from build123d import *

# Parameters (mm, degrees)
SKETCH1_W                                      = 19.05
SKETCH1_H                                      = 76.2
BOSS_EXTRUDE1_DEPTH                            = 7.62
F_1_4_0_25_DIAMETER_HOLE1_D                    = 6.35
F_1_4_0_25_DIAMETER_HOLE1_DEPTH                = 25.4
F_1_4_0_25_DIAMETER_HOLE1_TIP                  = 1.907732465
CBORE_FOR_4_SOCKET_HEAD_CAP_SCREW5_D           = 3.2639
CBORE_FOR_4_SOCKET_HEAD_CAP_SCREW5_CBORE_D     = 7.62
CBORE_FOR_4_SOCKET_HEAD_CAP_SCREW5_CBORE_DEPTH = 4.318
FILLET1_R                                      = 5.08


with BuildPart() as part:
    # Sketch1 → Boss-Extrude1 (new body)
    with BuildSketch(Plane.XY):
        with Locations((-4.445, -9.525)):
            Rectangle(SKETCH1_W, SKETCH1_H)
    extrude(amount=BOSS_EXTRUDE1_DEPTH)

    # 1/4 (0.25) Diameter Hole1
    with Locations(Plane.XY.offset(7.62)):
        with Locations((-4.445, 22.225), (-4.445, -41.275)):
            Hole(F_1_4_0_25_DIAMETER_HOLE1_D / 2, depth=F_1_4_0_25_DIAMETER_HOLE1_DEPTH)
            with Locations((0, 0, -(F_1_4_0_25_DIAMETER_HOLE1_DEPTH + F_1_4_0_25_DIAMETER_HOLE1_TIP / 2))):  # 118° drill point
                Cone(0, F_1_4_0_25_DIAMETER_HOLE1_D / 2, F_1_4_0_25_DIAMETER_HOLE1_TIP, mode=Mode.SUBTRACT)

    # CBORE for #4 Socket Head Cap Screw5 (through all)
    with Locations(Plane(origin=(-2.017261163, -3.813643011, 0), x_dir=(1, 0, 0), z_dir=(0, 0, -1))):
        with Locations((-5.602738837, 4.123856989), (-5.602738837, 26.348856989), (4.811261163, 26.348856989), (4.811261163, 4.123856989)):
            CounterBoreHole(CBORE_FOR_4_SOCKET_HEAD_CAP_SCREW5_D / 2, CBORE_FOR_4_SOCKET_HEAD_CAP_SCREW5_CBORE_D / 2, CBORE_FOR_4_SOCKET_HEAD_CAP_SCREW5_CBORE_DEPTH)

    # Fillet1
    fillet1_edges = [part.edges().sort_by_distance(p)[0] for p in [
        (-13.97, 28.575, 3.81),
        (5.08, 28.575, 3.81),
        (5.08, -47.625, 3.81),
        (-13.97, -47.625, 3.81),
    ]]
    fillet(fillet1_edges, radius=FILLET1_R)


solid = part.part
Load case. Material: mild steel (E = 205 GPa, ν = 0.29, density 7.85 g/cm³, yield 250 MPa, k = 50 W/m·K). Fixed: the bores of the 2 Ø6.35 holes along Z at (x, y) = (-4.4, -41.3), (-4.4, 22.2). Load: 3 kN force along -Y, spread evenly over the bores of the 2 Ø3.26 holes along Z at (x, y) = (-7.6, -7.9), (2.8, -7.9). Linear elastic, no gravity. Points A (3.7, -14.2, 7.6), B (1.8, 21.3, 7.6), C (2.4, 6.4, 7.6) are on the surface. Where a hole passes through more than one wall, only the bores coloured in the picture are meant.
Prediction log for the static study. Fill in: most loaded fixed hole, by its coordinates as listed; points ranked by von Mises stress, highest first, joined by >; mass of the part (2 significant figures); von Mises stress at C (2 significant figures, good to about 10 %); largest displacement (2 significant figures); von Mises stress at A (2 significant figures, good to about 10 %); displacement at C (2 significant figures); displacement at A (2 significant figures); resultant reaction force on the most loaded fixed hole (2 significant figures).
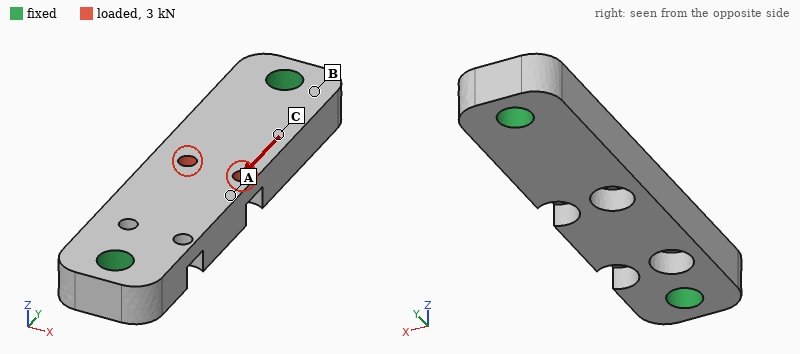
(-4.4, 22.2)
A > C > B
75 g
22 MPa
3.9 µm
35 MPa
1.2 µm
2.9 µm
1.7 kN
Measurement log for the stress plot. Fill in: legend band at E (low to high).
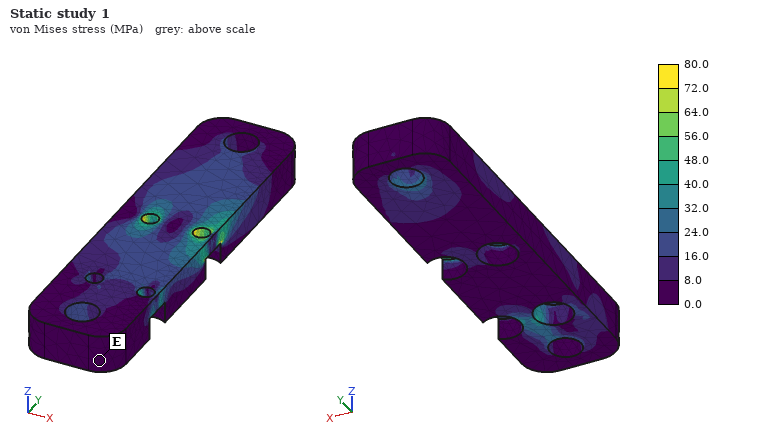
0.0 to 8.0 MPa
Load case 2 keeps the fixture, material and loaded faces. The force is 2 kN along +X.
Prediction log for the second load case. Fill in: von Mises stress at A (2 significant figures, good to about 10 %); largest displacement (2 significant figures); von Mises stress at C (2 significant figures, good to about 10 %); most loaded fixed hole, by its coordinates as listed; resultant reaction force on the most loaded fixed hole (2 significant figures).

28 MPa
14 µm
19 MPa
(-4.4, 22.2)
1.1 kN
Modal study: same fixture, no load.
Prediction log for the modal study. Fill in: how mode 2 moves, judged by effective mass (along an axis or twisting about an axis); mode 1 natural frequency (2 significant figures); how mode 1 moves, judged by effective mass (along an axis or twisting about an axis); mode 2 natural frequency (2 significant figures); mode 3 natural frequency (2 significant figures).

along X
9200 Hz
along Z
14 kHz
16 kHz
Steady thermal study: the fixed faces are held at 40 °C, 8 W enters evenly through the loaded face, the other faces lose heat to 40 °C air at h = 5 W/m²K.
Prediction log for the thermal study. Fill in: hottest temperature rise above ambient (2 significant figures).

28 K
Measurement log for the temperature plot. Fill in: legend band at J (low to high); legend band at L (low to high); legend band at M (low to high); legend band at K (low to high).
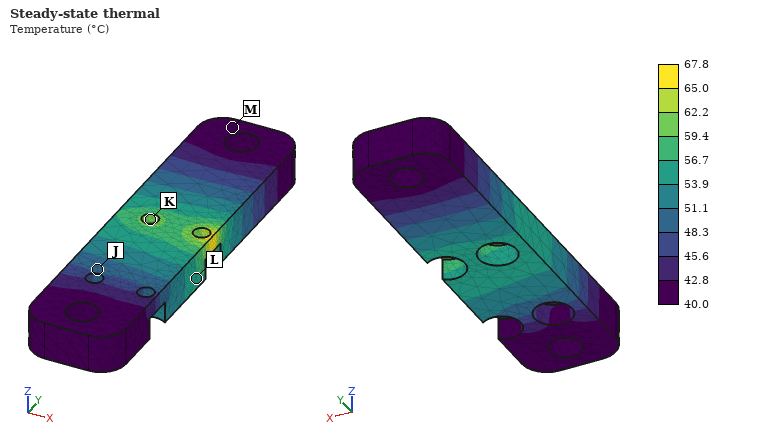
48.3 to 51.1 °C
53.9 to 56.7 °C
40.0 to 42.8 °C
59.4 to 62.2 °C
